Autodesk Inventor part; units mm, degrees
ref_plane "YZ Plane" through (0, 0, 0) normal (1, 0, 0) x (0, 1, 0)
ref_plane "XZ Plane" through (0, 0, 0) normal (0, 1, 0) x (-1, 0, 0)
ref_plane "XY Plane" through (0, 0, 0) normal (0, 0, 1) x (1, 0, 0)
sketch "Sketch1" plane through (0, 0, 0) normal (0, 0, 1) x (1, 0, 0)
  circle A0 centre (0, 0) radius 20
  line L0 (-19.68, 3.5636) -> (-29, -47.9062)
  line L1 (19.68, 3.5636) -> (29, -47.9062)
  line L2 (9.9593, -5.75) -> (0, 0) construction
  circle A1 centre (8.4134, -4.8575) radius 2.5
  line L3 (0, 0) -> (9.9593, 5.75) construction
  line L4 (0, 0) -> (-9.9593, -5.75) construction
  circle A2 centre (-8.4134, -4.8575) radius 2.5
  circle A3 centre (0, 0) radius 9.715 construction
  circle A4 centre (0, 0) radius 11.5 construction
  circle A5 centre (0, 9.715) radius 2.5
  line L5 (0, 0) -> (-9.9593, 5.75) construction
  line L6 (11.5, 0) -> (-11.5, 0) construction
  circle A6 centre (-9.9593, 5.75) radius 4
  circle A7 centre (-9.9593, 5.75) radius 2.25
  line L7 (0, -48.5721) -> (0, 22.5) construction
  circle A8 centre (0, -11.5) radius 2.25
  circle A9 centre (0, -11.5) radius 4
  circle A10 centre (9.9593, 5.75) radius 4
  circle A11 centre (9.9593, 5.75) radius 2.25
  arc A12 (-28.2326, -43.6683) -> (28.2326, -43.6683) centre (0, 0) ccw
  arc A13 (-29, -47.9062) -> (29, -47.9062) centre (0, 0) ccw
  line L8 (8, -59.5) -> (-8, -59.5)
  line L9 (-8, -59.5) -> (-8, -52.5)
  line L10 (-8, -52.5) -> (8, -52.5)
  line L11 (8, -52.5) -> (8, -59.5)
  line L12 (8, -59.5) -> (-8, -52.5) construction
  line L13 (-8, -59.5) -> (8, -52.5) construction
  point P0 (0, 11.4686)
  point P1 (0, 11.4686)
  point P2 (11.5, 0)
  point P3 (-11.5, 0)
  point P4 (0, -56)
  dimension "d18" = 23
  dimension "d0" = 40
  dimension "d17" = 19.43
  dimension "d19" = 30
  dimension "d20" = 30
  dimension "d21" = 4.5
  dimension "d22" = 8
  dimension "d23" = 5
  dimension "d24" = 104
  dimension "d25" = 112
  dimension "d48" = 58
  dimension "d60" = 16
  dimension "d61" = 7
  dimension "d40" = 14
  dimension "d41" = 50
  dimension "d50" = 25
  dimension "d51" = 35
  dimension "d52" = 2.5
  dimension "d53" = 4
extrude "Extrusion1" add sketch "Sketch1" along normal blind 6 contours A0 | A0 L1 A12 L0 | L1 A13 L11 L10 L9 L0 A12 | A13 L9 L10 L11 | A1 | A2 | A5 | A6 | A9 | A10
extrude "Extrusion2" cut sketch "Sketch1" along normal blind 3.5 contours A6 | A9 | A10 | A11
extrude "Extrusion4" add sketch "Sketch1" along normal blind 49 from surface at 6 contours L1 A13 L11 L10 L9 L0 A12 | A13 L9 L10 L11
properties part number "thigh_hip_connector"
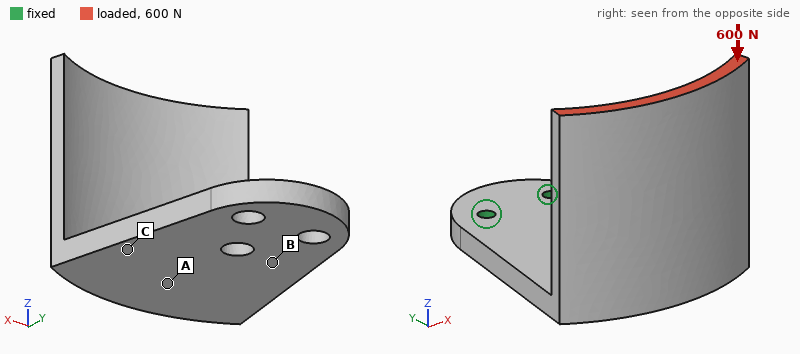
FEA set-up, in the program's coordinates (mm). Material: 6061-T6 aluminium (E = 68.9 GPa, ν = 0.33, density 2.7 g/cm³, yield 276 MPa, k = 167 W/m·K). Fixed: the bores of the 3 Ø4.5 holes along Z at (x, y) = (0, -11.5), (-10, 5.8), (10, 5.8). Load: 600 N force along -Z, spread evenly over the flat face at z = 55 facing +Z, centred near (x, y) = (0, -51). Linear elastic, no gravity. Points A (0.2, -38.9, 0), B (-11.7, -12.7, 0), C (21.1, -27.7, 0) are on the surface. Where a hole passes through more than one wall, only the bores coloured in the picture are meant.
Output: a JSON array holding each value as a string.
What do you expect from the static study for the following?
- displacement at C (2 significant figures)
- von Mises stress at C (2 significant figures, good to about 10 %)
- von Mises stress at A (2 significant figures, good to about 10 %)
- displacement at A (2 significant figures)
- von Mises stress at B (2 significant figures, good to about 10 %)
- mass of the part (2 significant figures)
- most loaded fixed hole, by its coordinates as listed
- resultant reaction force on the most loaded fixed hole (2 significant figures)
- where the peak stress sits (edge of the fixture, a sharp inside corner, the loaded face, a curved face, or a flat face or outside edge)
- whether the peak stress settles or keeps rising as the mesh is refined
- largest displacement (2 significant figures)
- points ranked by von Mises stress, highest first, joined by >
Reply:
["0.10 mm", "46 MPa", "20 MPa", "0.20 mm", "74 MPa", "84 g", "(0, -11.5)", "2.2 kN", "edge of the fixture", "keeps rising", "0.63 mm", "B > C > A"]
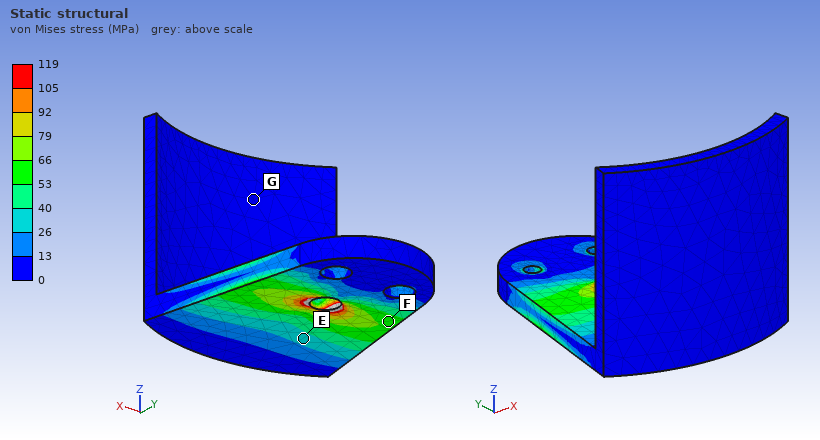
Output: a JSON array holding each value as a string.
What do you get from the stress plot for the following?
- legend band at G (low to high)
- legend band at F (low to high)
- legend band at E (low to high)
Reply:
["0 to 13 MPa", "53 to 66 MPa", "26 to 40 MPa"]
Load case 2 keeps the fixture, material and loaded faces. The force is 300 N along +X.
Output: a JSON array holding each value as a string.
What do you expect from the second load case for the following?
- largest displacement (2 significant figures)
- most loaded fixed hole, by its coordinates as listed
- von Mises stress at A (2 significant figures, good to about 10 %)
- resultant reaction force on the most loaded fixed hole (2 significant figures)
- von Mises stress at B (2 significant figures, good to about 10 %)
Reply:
["0.52 mm", "(0, -11.5)", "33 MPa", "1.2 kN", "45 MPa"]
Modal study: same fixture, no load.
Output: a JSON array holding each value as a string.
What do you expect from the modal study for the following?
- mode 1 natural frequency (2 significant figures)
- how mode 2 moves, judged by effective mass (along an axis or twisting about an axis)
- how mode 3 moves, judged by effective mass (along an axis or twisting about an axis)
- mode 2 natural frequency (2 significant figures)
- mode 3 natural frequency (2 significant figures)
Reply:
["750 Hz", "along X", "along Z", "1000 Hz", "1800 Hz"]
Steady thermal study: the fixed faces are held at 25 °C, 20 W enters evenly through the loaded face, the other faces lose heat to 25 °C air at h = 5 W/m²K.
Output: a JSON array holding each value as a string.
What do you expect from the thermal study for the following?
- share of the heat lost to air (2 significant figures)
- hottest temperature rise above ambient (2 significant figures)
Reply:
["6.7 %", "43 K"]
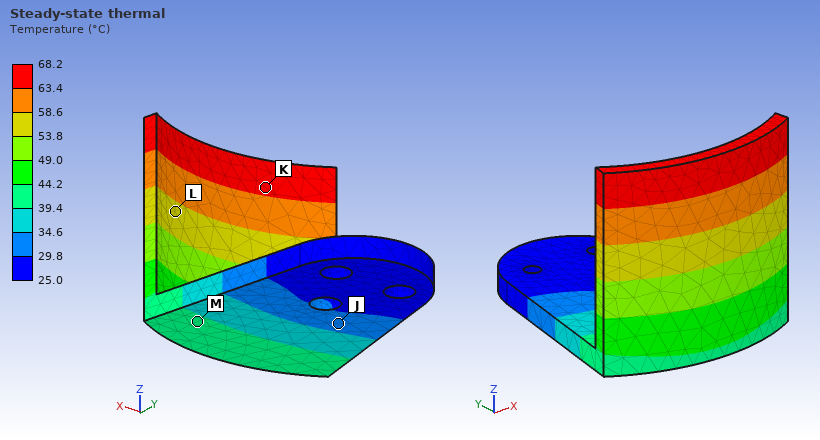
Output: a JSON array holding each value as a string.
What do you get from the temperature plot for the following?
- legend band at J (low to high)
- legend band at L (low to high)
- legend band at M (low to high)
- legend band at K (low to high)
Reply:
["29.8 to 34.6 °C", "53.8 to 58.6 °C", "39.4 to 44.2 °C", "63.4 to 68.2 °C"]
